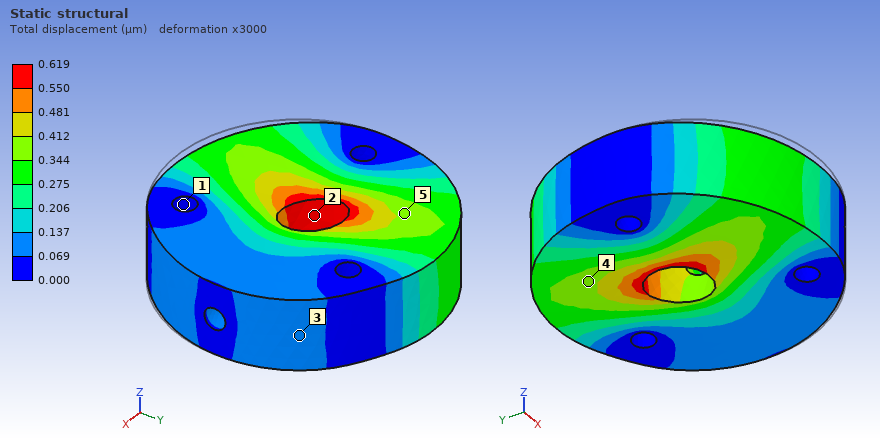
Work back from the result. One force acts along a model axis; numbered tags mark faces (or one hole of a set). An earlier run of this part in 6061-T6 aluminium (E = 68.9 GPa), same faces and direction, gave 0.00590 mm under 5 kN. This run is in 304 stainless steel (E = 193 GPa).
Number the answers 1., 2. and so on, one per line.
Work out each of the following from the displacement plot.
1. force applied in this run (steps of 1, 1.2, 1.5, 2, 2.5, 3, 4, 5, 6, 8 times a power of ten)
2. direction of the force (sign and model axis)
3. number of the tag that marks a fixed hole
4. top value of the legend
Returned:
1. 1.5 kN
2. +Y
3. 1
4. 0.619 µm
